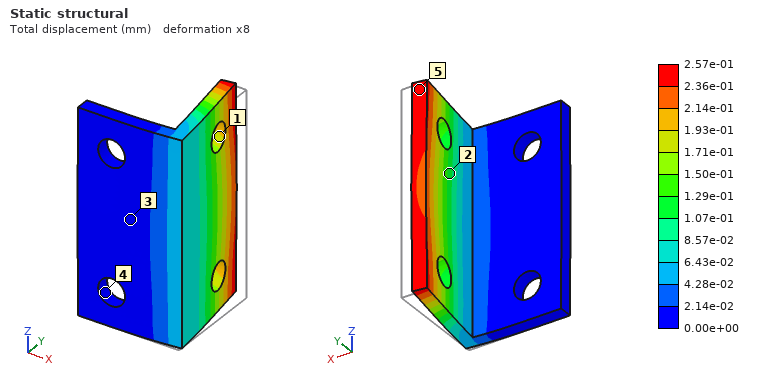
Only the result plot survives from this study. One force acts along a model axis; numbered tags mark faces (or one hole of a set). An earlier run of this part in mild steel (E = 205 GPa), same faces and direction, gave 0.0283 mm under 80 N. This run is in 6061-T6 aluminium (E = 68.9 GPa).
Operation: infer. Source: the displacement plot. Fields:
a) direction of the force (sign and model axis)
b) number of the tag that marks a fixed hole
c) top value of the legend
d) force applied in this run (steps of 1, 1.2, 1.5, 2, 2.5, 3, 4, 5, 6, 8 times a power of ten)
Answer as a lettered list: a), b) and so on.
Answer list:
a) -X
b) 4
c) 2.57e-01 mm
d) 250 N
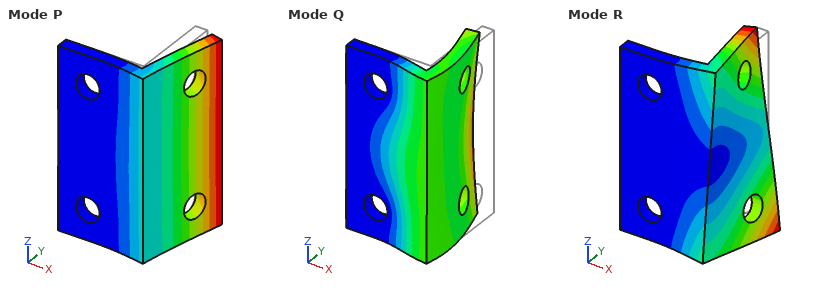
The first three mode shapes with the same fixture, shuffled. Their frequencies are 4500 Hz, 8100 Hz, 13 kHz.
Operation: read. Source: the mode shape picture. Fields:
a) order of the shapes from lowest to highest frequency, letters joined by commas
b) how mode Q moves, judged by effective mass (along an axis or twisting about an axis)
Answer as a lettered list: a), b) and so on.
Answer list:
a) P, R, Q
b) along Y
